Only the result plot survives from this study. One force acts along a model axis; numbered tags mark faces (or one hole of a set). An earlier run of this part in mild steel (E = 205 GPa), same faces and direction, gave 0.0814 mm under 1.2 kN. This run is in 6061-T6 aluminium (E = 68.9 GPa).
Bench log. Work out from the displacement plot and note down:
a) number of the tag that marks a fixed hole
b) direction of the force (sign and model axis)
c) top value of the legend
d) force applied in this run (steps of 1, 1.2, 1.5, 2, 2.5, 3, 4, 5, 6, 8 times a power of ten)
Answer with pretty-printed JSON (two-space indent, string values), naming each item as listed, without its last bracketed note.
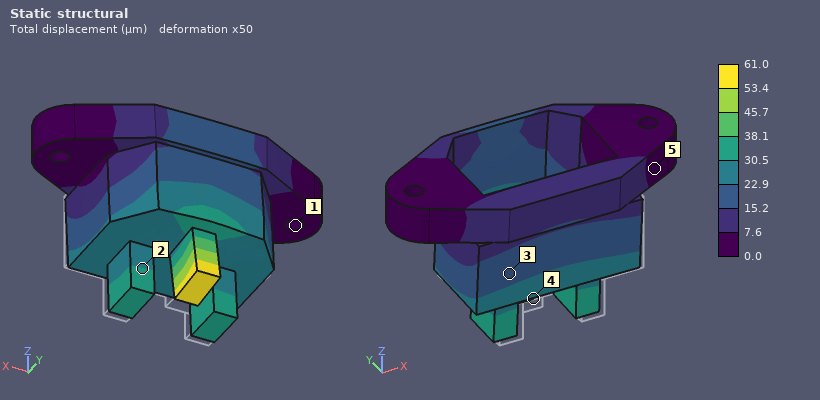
{
  "number of the tag that marks a fixed hole": "1",
  "direction of the force": "+Y",
  "top value of the legend": "61.0 µm",
  "force applied in this run": "300 N"
}
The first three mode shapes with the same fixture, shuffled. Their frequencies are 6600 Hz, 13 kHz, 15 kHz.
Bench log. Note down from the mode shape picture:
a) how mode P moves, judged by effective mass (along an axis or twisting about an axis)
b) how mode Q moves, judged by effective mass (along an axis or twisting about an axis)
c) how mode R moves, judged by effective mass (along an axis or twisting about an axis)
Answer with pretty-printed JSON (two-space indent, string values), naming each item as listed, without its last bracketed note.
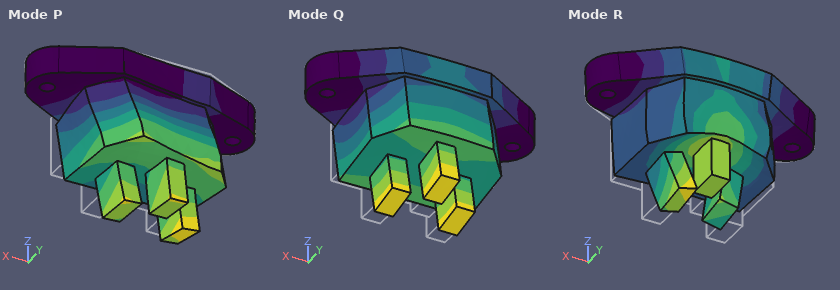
{
  "how mode P moves, judged by effective mass": "along X",
  "how mode Q moves, judged by effective mass": "along Y",
  "how mode R moves, judged by effective mass": "along Z"
}
